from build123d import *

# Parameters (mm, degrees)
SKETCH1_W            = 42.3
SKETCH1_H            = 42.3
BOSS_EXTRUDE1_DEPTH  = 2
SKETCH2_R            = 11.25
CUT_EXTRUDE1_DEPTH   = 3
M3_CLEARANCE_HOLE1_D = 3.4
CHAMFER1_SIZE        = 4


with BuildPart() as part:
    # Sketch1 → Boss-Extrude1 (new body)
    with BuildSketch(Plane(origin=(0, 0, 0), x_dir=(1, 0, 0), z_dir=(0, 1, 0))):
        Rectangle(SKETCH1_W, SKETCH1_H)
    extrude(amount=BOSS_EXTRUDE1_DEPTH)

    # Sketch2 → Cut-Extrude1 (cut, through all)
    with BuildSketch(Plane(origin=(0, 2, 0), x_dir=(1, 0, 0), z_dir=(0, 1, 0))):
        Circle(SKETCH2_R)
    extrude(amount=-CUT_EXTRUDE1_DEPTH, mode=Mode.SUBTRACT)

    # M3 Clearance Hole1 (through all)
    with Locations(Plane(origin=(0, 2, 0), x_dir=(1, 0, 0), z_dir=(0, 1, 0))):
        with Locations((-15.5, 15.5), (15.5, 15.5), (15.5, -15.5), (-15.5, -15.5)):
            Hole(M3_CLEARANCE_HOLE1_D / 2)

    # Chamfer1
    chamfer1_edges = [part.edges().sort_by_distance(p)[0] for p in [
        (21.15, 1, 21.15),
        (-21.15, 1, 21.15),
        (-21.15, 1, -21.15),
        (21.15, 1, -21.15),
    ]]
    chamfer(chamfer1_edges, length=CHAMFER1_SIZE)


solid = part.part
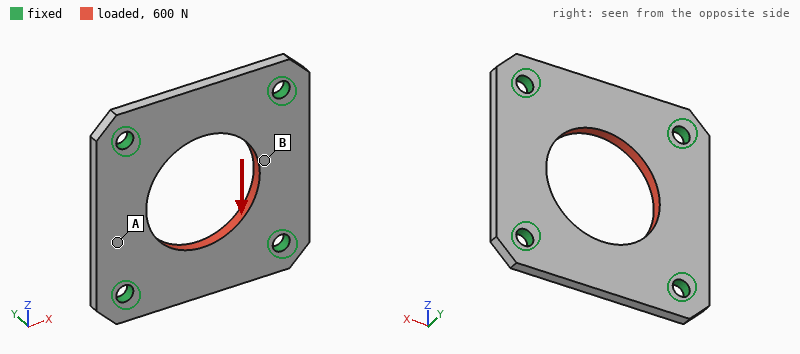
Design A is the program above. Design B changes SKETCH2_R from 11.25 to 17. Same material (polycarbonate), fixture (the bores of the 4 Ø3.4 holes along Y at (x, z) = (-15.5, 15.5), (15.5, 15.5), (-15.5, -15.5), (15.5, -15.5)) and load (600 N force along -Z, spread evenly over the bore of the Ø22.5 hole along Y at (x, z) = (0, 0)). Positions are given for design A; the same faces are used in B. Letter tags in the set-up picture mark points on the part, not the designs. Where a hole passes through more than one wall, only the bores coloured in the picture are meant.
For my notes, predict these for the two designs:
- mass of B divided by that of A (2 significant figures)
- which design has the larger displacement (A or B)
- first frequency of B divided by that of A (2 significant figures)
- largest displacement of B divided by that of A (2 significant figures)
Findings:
0.61
B
1.1
2.0
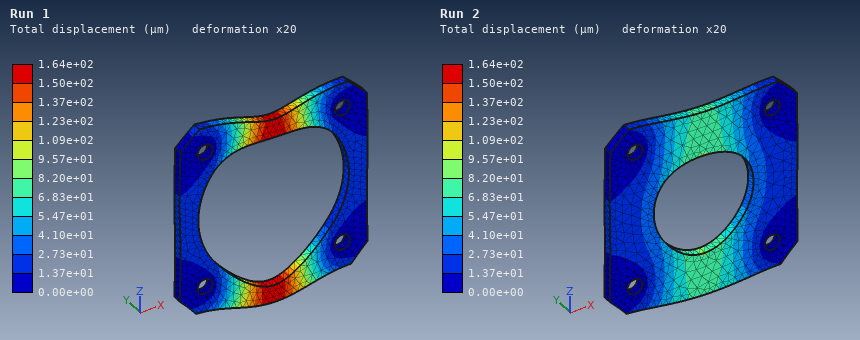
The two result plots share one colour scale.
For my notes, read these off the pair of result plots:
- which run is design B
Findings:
Run 1
